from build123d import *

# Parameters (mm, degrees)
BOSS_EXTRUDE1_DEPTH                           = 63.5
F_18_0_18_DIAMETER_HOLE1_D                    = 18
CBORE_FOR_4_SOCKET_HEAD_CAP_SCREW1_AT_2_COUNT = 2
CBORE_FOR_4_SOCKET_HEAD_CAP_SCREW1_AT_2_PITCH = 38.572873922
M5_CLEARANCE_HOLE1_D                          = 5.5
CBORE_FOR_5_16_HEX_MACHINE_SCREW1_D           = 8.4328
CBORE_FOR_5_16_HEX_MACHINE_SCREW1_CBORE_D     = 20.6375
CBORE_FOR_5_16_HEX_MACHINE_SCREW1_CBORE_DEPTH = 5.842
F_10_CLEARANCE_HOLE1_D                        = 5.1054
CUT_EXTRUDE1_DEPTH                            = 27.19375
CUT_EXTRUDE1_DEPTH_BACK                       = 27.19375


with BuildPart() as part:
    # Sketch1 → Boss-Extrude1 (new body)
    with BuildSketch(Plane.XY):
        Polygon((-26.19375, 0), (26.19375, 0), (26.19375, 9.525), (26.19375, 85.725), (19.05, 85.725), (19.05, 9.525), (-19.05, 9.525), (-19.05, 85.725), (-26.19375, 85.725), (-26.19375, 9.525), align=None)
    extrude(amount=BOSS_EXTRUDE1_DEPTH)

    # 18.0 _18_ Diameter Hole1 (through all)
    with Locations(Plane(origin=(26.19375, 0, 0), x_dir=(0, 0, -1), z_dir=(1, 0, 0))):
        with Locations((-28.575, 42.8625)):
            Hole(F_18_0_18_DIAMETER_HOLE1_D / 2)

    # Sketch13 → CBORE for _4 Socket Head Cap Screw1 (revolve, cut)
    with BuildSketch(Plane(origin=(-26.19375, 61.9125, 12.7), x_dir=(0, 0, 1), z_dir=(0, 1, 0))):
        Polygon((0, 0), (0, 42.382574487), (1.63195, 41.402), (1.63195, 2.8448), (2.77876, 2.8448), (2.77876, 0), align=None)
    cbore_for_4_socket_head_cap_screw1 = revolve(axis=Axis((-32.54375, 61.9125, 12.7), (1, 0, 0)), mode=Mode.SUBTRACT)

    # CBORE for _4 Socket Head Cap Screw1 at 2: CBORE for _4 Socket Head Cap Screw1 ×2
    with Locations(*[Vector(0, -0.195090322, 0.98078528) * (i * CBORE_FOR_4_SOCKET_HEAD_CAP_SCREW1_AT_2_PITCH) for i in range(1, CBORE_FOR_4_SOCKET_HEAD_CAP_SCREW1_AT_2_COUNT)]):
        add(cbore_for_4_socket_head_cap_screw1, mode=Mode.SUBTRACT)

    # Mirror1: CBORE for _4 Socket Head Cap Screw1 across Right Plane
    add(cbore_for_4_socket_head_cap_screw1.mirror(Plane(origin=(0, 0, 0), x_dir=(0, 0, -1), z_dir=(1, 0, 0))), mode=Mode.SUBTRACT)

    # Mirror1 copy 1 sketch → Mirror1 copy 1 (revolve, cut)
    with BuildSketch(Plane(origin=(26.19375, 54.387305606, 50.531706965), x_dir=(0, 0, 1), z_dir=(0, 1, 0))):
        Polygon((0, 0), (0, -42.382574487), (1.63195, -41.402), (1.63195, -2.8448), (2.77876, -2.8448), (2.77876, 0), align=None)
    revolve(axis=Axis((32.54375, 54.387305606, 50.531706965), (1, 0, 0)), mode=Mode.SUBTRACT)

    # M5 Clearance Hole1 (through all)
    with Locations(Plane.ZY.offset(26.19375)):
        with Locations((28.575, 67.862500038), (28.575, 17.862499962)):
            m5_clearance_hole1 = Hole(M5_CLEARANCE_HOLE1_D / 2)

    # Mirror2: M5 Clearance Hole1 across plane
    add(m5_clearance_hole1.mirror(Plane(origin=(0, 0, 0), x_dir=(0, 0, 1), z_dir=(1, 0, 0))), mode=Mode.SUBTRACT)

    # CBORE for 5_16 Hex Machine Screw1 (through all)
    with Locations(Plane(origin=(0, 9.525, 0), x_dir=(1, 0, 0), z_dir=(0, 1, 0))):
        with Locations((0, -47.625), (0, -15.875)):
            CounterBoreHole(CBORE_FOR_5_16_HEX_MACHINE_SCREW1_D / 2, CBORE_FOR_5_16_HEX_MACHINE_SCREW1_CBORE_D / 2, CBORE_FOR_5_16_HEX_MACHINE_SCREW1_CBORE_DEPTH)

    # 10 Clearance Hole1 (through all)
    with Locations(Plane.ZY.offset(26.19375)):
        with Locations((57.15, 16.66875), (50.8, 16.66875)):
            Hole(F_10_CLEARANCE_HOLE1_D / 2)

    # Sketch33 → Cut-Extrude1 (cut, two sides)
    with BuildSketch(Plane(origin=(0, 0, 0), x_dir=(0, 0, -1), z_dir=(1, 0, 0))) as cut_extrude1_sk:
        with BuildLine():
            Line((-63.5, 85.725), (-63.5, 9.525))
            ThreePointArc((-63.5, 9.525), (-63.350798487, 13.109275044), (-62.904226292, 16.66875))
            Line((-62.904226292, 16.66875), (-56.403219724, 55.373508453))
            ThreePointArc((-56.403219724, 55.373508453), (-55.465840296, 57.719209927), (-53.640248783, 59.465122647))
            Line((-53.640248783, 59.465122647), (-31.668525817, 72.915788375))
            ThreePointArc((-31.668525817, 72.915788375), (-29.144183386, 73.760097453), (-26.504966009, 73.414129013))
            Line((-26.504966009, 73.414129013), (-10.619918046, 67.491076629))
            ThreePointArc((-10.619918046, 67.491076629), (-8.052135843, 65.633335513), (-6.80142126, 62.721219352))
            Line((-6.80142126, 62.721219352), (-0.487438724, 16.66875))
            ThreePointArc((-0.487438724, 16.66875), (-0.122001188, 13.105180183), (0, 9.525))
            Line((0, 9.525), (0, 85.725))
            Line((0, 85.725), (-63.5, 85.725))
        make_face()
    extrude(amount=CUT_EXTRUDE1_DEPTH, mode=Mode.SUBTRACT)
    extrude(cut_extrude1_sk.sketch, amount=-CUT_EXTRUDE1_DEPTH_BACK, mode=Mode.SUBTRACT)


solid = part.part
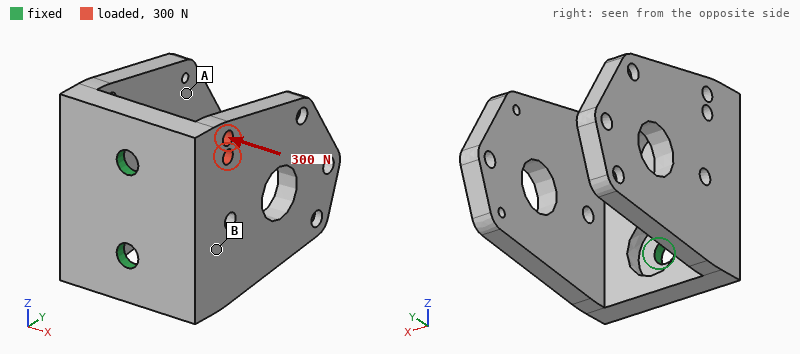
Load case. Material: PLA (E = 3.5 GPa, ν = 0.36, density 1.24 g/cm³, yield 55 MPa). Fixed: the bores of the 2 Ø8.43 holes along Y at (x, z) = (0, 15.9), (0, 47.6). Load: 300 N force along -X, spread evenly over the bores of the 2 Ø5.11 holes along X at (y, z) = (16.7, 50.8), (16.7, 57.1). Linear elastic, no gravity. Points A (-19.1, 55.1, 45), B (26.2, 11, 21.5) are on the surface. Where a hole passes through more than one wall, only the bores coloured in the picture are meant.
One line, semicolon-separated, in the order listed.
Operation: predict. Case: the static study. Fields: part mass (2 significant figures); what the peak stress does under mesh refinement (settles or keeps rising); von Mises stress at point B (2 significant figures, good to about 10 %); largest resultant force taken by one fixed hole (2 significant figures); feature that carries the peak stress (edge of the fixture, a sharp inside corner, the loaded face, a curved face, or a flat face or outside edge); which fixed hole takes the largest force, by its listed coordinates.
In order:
85 g; keeps rising; 3.0 MPa; 330 N; edge of the fixture; (0, 47.6)
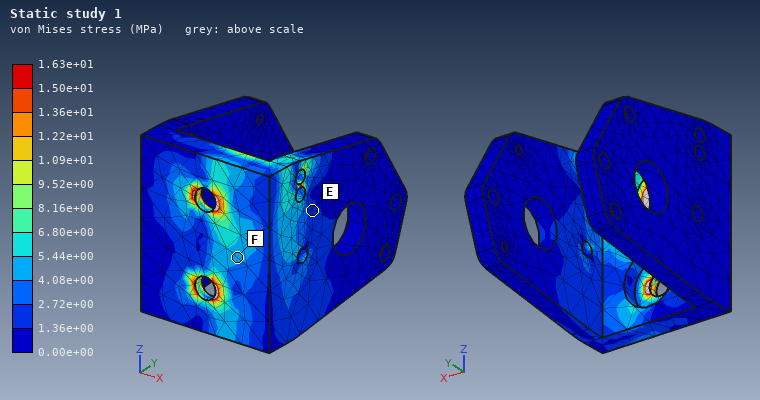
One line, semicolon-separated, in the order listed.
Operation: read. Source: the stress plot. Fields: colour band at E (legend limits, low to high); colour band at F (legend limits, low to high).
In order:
1.36e+00 to 2.72e+00 MPa; 4.08e+00 to 5.44e+00 MPa
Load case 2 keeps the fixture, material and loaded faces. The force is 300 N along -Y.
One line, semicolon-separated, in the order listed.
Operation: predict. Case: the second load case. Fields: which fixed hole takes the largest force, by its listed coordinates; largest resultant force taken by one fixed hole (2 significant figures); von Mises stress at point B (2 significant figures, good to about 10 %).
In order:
(0, 47.6); 330 N; 2.6 MPa
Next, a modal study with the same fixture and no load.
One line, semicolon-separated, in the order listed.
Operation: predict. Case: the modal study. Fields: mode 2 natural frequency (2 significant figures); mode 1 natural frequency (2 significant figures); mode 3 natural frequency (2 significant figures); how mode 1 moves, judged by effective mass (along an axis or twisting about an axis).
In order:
420 Hz; 300 Hz; 770 Hz; along X
